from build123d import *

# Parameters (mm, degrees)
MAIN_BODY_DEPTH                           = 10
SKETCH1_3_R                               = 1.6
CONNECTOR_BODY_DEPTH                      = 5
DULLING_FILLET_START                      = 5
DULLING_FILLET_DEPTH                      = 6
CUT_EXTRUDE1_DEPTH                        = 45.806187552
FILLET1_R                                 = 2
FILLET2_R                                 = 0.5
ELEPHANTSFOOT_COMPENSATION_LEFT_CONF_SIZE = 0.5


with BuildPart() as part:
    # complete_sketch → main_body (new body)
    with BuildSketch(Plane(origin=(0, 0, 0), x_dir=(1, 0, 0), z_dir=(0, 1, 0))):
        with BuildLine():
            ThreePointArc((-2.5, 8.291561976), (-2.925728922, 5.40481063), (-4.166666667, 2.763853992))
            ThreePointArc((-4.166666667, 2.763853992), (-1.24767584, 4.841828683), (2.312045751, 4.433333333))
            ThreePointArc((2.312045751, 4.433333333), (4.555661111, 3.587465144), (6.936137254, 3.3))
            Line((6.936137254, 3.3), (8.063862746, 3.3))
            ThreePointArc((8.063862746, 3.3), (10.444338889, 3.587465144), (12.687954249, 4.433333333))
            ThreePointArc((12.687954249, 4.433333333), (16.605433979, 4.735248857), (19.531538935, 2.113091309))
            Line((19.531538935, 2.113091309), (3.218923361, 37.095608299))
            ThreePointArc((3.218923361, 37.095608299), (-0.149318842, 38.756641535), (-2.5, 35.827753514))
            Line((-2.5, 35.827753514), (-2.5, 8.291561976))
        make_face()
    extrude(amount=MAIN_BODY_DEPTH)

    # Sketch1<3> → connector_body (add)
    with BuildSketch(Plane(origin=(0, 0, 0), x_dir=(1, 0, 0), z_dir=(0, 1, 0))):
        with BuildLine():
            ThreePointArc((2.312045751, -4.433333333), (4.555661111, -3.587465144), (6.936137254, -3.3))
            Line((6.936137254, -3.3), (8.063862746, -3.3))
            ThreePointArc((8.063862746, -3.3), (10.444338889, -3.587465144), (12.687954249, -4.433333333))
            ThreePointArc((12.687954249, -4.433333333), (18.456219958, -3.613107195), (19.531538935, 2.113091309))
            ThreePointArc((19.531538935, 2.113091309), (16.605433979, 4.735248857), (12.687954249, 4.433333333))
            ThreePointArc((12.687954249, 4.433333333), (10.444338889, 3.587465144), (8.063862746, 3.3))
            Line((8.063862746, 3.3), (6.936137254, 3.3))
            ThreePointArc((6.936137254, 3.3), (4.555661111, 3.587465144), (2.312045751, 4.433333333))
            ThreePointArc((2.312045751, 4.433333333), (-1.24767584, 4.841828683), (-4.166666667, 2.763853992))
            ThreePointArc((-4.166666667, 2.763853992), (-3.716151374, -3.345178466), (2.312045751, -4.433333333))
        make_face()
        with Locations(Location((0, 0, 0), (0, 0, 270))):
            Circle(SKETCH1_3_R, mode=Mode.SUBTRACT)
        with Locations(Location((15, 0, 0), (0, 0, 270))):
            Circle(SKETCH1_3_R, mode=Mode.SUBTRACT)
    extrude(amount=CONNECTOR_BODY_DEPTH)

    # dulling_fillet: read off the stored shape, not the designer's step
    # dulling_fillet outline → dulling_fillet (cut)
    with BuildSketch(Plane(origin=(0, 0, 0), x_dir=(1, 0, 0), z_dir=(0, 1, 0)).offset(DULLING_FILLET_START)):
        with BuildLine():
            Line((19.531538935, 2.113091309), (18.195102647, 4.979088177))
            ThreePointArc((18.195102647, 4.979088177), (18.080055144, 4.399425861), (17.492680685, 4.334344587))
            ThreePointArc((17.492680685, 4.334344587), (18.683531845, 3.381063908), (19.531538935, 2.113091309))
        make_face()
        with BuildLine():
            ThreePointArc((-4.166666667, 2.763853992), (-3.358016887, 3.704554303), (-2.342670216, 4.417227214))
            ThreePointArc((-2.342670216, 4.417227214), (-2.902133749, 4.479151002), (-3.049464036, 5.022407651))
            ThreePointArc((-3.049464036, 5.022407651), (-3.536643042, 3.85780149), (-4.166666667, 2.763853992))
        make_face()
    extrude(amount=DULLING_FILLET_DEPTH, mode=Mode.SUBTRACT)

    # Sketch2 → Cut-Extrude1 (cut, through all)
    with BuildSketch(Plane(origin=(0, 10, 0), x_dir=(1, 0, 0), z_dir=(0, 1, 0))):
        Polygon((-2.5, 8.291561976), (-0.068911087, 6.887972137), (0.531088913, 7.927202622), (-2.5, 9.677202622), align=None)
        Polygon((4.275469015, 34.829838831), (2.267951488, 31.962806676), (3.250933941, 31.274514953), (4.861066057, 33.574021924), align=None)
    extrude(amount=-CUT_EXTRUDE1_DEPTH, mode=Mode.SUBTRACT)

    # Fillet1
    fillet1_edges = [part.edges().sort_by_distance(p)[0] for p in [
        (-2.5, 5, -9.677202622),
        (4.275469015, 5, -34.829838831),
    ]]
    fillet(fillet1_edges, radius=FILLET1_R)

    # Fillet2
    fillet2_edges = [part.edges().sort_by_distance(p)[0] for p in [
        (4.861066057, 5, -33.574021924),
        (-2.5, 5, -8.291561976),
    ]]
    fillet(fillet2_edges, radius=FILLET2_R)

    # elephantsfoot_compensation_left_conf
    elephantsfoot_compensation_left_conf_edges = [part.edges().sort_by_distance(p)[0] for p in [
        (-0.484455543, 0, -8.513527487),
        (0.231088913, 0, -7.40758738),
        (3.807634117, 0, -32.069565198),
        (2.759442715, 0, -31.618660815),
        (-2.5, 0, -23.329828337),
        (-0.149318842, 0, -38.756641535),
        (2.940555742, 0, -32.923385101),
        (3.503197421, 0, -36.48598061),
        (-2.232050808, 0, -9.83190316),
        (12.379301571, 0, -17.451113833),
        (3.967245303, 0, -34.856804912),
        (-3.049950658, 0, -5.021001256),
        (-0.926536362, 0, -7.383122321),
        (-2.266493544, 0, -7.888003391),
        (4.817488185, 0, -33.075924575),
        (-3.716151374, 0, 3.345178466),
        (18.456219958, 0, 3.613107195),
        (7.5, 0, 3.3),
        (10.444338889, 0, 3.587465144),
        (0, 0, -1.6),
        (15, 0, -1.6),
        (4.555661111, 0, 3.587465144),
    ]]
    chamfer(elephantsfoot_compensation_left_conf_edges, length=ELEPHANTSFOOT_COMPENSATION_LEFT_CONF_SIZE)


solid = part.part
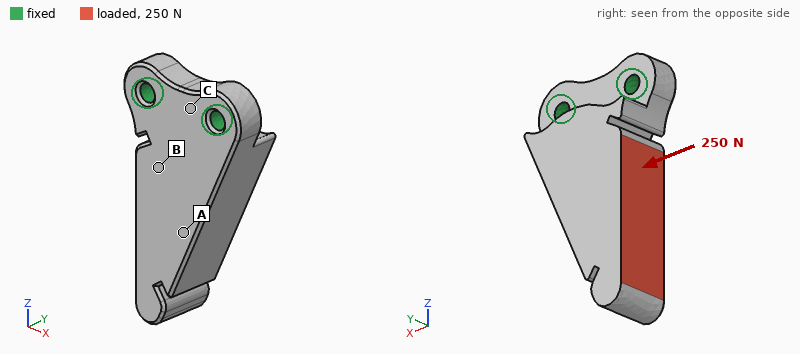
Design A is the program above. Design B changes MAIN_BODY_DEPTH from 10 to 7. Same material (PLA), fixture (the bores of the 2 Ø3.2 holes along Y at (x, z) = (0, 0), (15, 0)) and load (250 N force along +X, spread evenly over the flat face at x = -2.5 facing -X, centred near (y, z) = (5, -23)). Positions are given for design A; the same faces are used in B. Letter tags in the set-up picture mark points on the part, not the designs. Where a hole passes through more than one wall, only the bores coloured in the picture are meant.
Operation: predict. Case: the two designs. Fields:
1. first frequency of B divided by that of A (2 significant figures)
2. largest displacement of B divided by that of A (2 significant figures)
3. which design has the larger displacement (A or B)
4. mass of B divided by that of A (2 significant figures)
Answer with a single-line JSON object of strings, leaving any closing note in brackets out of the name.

{"first frequency of B divided by that of A": "1.1", "largest displacement of B divided by that of A": "1.2", "which design has the larger displacement": "B", "mass of B divided by that of A": "0.75"}
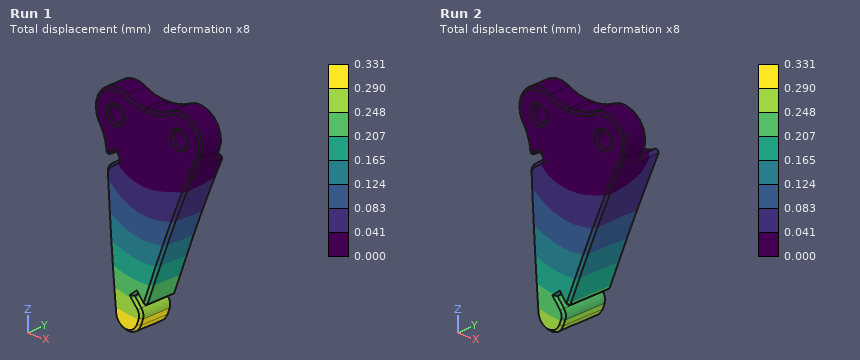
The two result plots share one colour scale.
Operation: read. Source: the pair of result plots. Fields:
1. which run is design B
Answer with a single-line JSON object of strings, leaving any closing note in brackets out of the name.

{"which run is design B": "Run 1"}
